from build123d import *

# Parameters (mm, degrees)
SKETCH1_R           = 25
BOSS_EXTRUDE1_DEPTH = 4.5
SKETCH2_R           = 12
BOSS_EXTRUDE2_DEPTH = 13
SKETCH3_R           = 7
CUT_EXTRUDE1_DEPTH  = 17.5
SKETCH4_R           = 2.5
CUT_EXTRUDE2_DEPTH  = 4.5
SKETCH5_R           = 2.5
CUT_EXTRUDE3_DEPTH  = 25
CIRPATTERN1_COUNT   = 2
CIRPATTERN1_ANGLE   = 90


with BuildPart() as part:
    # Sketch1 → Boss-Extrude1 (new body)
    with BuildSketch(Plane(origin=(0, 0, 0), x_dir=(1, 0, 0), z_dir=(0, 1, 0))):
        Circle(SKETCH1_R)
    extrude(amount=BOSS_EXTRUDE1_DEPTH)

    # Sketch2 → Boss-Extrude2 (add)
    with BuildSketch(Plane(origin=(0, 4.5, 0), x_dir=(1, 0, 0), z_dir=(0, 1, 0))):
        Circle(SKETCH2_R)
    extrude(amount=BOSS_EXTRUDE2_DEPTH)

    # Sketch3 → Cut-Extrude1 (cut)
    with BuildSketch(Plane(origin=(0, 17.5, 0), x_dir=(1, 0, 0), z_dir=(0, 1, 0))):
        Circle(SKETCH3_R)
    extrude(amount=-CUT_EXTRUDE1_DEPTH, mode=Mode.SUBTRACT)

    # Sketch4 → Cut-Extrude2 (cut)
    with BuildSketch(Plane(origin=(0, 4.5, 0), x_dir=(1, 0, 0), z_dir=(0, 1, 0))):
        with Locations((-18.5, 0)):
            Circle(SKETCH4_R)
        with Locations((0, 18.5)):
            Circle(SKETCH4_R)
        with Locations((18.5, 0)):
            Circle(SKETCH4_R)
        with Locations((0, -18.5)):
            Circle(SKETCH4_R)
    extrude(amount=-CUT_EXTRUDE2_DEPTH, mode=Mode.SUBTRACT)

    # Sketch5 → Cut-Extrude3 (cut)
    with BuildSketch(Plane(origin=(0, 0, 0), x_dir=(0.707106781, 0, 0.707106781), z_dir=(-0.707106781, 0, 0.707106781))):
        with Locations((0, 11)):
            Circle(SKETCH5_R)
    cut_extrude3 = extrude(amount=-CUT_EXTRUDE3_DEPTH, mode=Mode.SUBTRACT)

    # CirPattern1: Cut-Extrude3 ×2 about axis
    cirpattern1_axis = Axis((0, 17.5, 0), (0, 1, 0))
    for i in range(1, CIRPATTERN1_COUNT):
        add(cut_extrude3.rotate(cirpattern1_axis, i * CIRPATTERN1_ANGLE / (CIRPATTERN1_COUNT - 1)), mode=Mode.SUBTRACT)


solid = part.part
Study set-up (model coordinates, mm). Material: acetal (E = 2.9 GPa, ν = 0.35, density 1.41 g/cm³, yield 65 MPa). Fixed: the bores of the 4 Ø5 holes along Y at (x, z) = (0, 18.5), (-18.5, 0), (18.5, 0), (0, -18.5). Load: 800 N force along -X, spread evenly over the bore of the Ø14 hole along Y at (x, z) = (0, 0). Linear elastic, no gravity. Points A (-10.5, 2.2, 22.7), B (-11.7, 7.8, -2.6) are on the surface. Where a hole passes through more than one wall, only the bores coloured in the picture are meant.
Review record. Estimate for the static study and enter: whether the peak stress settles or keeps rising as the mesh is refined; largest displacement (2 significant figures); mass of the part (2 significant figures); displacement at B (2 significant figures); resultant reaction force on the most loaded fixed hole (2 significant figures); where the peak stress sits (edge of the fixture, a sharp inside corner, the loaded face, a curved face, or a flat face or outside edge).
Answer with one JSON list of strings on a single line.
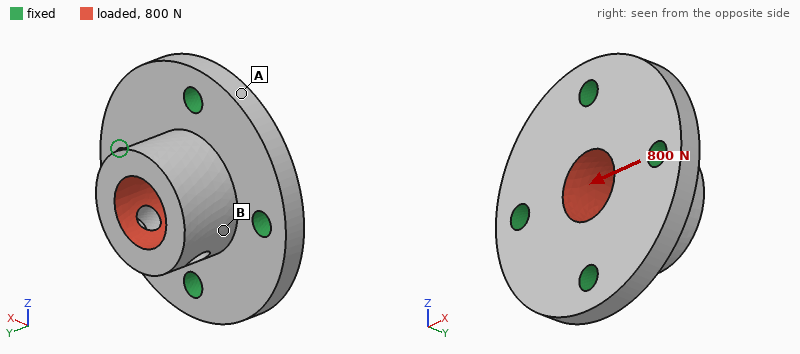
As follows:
["keeps rising", "83 µm", "16 g", "42 µm", "300 N", "edge of the fixture"]
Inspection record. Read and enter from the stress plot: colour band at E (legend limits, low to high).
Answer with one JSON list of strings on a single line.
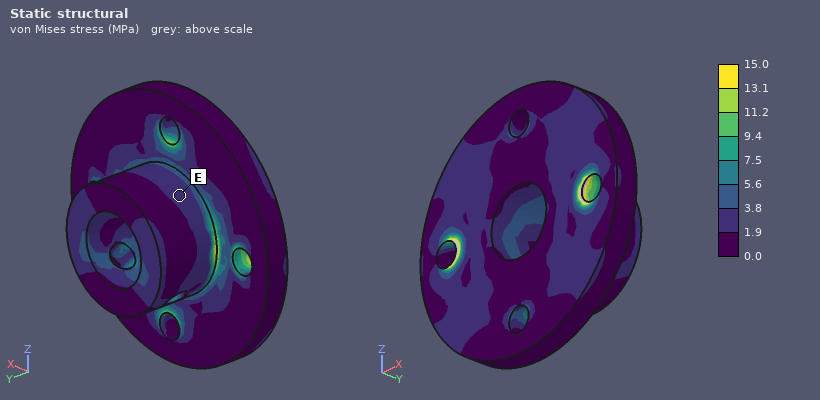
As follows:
["1.9 to 3.8 MPa"]
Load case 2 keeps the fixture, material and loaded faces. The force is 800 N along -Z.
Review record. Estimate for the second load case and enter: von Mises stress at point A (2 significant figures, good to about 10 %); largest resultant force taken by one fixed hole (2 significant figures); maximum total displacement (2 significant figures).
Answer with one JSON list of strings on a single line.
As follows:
["1.3 MPa", "300 N", "83 µm"]
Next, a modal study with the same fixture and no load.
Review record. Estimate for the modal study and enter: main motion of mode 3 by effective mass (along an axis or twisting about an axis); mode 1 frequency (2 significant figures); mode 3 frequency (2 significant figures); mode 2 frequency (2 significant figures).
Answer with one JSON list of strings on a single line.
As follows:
["along Y", "6100 Hz", "6700 Hz", "6100 Hz"]
